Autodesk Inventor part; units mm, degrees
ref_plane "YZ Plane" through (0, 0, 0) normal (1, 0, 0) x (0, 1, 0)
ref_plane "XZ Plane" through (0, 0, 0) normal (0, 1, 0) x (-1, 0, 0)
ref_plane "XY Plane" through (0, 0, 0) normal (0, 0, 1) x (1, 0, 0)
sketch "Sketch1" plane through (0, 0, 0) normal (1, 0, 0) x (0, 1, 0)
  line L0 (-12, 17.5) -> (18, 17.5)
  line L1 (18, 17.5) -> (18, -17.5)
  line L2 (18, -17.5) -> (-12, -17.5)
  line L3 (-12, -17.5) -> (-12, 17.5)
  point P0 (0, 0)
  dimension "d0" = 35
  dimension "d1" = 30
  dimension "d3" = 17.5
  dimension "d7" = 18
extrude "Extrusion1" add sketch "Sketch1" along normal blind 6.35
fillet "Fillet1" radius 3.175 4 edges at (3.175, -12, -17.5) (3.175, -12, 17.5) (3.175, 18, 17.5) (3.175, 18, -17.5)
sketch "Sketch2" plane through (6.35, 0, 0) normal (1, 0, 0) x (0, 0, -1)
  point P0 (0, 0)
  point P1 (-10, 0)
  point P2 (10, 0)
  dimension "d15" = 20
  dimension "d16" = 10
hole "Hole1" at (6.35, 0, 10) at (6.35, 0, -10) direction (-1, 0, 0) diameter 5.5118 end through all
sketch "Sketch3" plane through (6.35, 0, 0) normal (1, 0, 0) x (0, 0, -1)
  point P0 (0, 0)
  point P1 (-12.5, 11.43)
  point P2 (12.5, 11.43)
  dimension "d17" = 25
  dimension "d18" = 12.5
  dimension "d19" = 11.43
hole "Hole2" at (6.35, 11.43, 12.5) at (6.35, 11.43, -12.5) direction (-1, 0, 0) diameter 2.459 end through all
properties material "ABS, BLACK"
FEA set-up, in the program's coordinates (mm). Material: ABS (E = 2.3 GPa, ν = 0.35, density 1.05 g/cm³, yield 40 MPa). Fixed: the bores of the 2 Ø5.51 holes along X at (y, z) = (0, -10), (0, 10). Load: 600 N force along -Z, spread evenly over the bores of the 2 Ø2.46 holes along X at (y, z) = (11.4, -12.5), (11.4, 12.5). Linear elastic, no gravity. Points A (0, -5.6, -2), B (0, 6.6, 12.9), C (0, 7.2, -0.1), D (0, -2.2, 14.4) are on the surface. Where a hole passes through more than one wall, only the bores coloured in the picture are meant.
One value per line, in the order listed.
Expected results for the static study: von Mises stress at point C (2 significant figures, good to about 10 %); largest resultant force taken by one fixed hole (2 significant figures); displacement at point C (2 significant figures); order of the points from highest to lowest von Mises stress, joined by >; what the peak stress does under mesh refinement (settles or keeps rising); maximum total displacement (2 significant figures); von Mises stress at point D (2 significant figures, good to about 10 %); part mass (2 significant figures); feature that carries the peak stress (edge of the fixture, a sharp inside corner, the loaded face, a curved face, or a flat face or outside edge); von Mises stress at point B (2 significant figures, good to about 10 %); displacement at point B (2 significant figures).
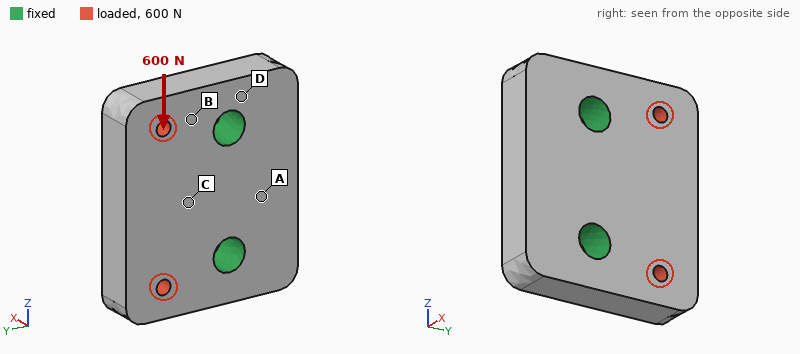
5.3 MPa
390 N
23 µm
C > B > D > A
keeps rising
62 µm
2.5 MPa
6.6 g
edge of the fixture
4.3 MPa
27 µm
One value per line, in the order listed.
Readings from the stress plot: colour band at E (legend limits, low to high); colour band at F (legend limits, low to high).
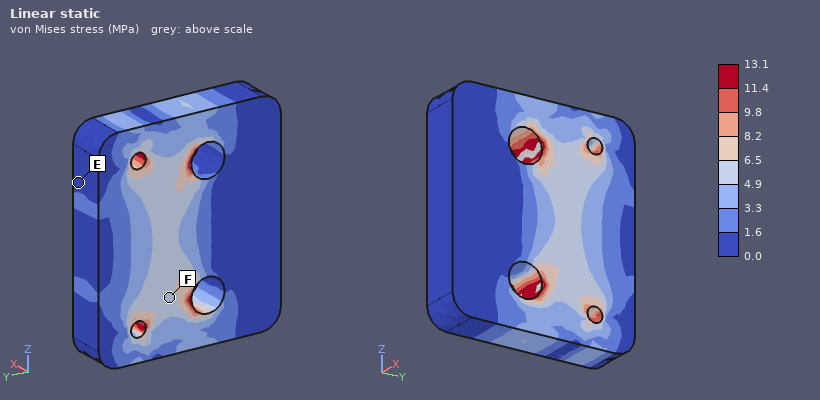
0.0 to 1.6 MPa
4.9 to 6.5 MPa
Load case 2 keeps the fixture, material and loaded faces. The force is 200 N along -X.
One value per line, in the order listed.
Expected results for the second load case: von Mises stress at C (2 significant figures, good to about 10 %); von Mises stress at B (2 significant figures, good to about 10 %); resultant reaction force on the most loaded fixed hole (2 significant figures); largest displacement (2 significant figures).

2.4 MPa
4.6 MPa
100 N
0.11 mm
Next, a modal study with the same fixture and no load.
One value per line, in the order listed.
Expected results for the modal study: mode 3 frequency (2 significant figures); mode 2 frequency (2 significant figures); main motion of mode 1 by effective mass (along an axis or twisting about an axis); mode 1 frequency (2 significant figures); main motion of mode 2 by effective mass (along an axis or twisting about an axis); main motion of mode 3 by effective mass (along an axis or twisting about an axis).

10 kHz
6900 Hz
along X
4800 Hz
twisting about Y
along X
